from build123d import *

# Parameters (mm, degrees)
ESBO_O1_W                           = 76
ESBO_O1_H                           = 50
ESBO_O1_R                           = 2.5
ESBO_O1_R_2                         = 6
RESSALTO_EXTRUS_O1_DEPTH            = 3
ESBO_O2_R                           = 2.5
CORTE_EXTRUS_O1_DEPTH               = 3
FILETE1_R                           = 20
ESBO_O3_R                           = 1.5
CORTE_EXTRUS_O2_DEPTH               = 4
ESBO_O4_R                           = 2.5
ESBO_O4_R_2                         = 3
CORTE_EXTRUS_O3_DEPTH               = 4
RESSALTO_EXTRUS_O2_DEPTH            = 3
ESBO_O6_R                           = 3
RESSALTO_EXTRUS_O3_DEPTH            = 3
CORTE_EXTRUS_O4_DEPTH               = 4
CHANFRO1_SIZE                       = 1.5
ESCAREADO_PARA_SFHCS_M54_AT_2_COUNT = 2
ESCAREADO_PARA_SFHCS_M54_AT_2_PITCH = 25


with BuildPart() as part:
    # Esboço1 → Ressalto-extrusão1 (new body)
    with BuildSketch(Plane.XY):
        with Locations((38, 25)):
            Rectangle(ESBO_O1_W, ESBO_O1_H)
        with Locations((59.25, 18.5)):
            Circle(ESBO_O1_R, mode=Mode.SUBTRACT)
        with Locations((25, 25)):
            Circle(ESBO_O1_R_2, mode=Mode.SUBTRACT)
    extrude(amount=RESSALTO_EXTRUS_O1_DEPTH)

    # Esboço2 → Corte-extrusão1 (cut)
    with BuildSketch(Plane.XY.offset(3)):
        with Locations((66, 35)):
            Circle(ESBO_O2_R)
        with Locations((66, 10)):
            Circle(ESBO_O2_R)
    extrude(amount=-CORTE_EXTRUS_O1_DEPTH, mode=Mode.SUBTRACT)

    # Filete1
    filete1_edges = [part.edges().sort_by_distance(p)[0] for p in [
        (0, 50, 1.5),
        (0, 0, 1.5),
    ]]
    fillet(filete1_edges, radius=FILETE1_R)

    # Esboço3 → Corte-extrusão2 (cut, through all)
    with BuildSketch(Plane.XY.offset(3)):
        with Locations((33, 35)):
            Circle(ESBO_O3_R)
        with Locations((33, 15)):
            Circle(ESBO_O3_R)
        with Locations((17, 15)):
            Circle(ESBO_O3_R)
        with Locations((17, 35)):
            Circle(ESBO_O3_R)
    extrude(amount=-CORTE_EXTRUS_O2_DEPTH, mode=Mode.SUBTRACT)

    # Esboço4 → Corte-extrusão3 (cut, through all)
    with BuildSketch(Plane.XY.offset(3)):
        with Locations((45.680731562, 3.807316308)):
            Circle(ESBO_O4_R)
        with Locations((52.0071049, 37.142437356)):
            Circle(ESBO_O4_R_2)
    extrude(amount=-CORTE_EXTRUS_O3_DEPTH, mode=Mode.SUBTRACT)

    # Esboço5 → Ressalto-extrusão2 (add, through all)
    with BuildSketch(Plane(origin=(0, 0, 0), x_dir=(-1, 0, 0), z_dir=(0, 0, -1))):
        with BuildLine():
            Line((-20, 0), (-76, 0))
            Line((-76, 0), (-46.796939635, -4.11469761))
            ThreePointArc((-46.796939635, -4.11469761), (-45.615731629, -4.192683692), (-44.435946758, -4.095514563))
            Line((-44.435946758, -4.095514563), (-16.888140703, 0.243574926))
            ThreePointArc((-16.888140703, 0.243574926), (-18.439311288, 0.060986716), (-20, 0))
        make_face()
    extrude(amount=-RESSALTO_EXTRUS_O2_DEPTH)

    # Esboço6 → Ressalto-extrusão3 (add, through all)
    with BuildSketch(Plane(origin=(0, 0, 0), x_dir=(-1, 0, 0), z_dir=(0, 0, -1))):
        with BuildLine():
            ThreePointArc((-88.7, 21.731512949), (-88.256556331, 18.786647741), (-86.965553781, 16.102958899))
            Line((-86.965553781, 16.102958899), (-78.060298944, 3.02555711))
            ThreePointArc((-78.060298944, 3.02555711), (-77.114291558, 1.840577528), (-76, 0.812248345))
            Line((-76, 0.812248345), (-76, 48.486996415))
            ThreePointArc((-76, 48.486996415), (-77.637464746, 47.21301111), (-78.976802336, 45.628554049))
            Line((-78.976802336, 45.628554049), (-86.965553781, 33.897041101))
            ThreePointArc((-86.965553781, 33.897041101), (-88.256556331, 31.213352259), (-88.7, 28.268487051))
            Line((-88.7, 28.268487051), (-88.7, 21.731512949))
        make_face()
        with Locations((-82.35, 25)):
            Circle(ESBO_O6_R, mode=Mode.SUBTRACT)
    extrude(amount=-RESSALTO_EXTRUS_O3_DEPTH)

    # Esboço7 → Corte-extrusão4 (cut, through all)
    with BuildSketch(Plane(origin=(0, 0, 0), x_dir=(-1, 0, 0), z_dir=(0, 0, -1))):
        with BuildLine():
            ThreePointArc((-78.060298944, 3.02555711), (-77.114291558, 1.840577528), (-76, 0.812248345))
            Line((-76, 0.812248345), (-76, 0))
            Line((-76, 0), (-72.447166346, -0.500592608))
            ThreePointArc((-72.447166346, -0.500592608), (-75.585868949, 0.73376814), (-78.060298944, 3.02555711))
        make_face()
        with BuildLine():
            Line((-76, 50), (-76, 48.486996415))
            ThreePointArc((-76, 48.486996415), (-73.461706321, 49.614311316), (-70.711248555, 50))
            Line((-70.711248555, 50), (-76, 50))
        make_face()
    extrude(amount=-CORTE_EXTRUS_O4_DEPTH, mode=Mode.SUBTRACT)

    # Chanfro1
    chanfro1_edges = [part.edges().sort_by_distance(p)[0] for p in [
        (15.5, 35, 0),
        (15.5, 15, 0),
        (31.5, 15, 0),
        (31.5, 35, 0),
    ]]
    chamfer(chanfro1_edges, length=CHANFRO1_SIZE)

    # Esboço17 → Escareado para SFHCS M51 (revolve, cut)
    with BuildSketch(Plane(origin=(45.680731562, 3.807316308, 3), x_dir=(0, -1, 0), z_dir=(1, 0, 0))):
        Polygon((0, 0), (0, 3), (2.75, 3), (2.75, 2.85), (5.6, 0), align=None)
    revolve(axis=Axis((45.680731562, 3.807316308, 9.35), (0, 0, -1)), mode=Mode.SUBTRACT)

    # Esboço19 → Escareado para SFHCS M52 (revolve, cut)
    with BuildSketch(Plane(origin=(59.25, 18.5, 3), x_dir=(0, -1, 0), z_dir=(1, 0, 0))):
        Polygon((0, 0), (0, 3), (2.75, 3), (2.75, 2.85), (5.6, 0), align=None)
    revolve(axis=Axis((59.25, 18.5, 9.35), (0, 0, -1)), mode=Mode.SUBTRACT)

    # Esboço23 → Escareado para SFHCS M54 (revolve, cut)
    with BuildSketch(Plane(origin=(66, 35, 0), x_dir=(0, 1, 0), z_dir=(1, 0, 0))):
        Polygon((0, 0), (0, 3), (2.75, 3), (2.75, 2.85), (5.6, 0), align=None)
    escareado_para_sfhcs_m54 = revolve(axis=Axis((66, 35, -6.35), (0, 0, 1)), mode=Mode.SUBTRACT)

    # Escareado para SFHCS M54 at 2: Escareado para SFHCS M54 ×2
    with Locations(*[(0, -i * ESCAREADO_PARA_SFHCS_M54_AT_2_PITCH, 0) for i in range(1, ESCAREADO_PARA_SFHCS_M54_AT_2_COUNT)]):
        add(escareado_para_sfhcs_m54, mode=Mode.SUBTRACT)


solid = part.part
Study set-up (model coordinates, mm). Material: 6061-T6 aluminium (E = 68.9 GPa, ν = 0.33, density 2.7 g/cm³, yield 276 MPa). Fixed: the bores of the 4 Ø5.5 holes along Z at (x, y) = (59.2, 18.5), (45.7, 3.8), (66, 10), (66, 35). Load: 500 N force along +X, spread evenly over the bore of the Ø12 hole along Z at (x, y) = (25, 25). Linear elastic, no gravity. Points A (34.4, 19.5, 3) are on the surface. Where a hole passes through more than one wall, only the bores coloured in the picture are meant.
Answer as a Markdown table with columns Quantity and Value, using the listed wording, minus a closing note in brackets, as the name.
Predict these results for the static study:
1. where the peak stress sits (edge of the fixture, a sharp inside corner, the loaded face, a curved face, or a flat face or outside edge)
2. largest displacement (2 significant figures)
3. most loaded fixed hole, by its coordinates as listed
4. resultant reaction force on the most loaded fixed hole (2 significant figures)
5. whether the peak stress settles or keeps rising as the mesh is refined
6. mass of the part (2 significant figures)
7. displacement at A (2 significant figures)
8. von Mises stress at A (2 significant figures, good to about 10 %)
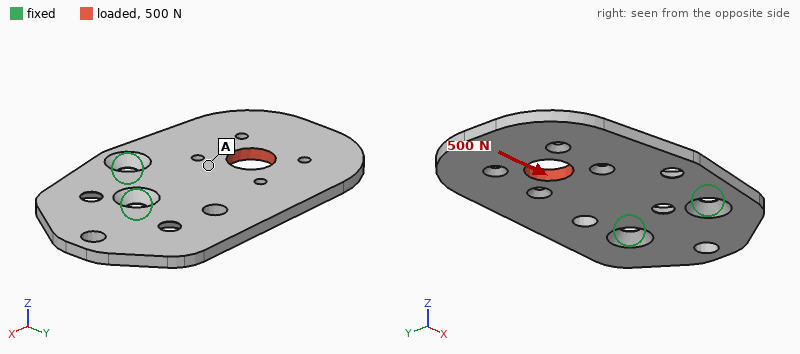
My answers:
| Quantity | Value |
|---|---|
| where the peak stress sits | edge of the fixture |
| largest displacement | 8.1 µm |
| most loaded fixed hole, by its coordinates as listed | (66, 35) |
| resultant reaction force on the most loaded fixed hole | 210 N |
| whether the peak stress settles or keeps rising as the mesh is refined | keeps rising |
| mass of the part | 30 g |
| displacement at A | 3.0 µm |
| von Mises stress at A | 5.8 MPa |
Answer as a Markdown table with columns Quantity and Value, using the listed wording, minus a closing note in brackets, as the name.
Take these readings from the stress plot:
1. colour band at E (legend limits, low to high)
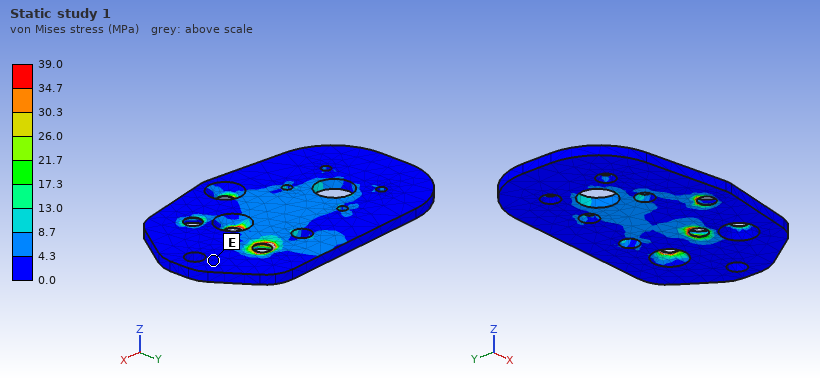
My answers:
| Quantity | Value |
|---|---|
| colour band at E | 0.0 to 4.3 MPa |
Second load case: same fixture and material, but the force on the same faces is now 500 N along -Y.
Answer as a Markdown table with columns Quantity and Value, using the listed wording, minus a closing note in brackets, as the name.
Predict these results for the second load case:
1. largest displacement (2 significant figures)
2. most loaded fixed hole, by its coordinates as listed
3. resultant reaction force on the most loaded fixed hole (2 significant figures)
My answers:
| Quantity | Value |
|---|---|
| largest displacement | 86 µm |
| most loaded fixed hole, by its coordinates as listed | (45.7, 3.8) |
| resultant reaction force on the most loaded fixed hole | 480 N |
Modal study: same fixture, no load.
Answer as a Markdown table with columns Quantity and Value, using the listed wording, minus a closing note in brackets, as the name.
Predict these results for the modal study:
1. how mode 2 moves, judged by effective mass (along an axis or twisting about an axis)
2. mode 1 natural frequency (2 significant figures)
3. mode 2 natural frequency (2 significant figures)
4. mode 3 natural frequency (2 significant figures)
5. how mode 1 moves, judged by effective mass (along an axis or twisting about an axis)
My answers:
| Quantity | Value |
|---|---|
| how mode 2 moves, judged by effective mass | twisting about X |
| mode 1 natural frequency | 760 Hz |
| mode 2 natural frequency | 2200 Hz |
| mode 3 natural frequency | 4000 Hz |
| how mode 1 moves, judged by effective mass | along Z |
